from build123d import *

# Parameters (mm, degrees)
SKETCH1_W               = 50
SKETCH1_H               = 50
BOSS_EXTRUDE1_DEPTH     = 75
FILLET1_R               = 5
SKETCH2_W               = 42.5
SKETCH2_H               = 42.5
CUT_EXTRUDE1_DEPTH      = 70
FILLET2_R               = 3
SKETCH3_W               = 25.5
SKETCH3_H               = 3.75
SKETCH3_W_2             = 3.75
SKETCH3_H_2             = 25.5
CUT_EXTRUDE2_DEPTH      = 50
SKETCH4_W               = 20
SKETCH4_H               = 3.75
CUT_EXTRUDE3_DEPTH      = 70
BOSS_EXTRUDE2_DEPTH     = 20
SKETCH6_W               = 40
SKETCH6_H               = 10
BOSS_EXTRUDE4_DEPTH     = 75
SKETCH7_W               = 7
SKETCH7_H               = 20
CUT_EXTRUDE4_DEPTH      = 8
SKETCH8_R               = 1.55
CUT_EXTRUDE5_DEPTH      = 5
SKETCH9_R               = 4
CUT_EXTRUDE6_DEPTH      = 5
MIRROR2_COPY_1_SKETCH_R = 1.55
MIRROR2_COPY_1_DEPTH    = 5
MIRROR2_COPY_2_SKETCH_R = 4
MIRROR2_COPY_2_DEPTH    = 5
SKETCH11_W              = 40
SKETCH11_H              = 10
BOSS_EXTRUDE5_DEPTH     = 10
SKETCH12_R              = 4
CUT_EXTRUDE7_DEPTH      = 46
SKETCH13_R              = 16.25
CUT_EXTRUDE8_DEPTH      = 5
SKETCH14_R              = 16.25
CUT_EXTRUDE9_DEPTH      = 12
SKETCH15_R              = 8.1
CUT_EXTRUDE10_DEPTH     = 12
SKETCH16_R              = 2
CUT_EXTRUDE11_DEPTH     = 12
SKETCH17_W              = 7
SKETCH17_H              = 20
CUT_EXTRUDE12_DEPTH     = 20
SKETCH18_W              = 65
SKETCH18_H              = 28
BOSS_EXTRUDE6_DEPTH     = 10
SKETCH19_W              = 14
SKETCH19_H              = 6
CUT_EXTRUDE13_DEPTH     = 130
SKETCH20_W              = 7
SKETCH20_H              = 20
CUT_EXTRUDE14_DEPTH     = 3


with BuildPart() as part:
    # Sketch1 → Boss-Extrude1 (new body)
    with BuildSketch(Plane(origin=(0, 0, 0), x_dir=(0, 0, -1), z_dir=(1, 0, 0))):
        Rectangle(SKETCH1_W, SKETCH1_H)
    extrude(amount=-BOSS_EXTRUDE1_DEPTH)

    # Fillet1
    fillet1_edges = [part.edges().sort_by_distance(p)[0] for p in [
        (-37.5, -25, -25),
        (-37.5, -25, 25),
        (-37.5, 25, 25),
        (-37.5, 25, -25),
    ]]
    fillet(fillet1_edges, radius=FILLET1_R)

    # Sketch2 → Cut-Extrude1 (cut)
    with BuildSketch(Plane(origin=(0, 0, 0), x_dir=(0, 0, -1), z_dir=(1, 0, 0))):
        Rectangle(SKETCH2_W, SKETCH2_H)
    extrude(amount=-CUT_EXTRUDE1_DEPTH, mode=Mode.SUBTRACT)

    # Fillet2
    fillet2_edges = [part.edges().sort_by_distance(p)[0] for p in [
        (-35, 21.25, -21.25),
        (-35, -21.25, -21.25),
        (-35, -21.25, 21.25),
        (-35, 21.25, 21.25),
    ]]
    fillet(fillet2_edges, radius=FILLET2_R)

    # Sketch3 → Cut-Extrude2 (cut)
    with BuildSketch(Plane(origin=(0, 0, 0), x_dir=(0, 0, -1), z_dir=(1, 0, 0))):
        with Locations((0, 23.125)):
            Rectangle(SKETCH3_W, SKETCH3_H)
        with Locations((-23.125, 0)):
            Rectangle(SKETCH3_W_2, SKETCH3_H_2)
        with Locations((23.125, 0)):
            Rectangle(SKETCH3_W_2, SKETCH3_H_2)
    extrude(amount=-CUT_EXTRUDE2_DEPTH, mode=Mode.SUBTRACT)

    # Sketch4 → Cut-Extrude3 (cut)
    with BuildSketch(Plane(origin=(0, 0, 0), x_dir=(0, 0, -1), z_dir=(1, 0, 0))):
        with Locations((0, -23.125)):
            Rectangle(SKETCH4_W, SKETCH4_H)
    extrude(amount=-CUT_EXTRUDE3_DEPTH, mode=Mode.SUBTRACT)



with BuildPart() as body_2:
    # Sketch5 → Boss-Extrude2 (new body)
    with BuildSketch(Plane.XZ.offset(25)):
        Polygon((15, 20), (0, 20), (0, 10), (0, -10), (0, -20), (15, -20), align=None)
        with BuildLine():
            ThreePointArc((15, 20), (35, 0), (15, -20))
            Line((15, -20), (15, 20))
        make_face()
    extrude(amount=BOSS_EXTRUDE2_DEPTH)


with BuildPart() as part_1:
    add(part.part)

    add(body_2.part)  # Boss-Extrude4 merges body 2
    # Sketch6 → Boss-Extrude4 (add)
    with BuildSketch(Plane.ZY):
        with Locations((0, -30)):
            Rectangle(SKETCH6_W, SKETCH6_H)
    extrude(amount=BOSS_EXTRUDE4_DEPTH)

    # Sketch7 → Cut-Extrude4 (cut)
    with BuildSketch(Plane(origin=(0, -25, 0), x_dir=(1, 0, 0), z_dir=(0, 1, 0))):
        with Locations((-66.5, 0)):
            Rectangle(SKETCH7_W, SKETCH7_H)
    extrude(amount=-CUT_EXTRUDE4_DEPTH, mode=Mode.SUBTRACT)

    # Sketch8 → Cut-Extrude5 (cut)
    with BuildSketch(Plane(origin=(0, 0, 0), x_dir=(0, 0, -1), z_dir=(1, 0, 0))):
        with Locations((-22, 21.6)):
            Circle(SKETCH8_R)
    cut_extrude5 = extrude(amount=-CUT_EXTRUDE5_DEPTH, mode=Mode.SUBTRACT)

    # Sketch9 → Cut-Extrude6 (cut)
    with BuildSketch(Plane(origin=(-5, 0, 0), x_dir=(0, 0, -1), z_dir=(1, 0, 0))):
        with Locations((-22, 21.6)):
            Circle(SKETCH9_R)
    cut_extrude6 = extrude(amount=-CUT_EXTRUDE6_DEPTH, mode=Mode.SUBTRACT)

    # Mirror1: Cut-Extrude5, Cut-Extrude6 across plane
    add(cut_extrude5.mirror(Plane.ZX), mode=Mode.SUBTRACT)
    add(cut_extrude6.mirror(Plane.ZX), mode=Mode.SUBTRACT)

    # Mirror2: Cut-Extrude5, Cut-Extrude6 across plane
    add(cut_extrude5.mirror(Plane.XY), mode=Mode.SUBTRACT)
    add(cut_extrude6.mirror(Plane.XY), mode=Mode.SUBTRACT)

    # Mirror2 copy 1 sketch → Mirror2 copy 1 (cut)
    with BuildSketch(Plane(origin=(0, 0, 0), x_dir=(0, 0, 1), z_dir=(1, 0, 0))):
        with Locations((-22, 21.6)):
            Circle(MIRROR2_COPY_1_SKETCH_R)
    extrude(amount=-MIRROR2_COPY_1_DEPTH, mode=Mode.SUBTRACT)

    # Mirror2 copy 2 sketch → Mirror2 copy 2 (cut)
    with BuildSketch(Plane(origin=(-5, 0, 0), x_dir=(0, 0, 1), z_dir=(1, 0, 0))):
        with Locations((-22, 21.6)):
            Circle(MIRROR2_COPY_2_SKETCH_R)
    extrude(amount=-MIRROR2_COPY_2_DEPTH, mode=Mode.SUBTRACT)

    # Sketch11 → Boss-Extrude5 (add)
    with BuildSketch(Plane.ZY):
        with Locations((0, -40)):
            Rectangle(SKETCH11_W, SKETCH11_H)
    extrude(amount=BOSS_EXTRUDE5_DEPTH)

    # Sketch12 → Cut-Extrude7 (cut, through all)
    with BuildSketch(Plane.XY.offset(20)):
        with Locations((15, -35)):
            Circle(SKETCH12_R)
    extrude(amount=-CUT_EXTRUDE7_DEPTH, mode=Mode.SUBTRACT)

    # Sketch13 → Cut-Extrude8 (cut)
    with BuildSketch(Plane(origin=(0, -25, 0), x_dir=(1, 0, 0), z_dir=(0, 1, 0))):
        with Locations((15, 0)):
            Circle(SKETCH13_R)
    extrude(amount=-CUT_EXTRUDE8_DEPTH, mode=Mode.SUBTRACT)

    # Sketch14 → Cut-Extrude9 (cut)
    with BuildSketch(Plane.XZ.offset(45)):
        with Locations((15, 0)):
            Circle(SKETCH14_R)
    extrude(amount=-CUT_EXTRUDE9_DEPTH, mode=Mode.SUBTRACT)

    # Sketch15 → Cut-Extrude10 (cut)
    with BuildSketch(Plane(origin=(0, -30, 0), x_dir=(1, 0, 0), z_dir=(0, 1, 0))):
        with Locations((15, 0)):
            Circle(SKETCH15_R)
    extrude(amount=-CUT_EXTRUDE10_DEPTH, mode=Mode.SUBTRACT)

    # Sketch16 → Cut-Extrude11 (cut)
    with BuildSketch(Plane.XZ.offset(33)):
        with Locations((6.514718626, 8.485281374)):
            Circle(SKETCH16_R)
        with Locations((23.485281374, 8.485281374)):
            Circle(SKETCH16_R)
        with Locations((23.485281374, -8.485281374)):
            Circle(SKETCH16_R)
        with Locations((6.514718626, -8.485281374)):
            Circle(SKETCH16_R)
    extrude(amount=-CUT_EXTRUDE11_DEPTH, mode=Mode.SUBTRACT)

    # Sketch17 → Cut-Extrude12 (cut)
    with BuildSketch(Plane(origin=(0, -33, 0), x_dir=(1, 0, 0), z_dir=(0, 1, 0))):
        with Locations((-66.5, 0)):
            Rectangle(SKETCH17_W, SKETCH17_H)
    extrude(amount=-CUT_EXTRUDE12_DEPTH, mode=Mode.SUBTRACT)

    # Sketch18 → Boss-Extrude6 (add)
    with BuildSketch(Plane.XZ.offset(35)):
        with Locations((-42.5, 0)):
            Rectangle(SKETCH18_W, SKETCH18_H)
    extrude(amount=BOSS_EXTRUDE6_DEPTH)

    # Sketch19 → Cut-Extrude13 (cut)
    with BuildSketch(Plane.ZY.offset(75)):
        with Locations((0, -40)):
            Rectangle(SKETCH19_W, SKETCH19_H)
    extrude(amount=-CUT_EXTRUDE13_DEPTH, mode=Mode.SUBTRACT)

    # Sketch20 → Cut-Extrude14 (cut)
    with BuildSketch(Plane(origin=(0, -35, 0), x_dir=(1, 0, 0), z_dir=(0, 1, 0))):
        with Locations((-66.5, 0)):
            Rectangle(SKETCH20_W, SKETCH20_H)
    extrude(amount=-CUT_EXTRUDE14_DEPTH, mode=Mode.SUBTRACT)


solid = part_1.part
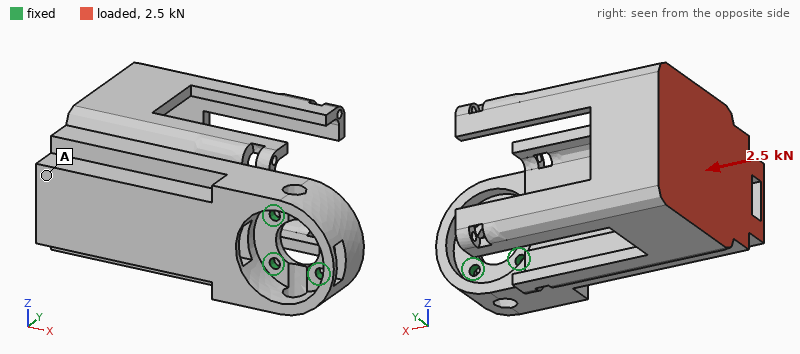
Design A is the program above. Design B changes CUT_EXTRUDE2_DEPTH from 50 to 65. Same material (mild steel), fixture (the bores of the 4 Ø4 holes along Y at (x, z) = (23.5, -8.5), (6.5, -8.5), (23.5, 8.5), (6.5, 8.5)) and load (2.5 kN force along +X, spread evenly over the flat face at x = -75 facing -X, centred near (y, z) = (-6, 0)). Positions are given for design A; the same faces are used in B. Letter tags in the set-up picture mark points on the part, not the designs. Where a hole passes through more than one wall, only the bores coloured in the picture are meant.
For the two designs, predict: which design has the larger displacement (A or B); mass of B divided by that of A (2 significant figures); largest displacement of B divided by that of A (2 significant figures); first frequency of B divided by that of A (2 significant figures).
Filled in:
B
0.95
1.4
1.0
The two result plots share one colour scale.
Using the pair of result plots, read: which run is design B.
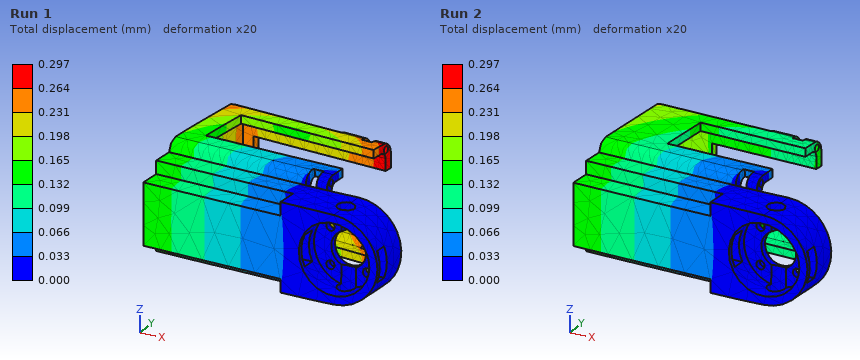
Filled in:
Run 1
